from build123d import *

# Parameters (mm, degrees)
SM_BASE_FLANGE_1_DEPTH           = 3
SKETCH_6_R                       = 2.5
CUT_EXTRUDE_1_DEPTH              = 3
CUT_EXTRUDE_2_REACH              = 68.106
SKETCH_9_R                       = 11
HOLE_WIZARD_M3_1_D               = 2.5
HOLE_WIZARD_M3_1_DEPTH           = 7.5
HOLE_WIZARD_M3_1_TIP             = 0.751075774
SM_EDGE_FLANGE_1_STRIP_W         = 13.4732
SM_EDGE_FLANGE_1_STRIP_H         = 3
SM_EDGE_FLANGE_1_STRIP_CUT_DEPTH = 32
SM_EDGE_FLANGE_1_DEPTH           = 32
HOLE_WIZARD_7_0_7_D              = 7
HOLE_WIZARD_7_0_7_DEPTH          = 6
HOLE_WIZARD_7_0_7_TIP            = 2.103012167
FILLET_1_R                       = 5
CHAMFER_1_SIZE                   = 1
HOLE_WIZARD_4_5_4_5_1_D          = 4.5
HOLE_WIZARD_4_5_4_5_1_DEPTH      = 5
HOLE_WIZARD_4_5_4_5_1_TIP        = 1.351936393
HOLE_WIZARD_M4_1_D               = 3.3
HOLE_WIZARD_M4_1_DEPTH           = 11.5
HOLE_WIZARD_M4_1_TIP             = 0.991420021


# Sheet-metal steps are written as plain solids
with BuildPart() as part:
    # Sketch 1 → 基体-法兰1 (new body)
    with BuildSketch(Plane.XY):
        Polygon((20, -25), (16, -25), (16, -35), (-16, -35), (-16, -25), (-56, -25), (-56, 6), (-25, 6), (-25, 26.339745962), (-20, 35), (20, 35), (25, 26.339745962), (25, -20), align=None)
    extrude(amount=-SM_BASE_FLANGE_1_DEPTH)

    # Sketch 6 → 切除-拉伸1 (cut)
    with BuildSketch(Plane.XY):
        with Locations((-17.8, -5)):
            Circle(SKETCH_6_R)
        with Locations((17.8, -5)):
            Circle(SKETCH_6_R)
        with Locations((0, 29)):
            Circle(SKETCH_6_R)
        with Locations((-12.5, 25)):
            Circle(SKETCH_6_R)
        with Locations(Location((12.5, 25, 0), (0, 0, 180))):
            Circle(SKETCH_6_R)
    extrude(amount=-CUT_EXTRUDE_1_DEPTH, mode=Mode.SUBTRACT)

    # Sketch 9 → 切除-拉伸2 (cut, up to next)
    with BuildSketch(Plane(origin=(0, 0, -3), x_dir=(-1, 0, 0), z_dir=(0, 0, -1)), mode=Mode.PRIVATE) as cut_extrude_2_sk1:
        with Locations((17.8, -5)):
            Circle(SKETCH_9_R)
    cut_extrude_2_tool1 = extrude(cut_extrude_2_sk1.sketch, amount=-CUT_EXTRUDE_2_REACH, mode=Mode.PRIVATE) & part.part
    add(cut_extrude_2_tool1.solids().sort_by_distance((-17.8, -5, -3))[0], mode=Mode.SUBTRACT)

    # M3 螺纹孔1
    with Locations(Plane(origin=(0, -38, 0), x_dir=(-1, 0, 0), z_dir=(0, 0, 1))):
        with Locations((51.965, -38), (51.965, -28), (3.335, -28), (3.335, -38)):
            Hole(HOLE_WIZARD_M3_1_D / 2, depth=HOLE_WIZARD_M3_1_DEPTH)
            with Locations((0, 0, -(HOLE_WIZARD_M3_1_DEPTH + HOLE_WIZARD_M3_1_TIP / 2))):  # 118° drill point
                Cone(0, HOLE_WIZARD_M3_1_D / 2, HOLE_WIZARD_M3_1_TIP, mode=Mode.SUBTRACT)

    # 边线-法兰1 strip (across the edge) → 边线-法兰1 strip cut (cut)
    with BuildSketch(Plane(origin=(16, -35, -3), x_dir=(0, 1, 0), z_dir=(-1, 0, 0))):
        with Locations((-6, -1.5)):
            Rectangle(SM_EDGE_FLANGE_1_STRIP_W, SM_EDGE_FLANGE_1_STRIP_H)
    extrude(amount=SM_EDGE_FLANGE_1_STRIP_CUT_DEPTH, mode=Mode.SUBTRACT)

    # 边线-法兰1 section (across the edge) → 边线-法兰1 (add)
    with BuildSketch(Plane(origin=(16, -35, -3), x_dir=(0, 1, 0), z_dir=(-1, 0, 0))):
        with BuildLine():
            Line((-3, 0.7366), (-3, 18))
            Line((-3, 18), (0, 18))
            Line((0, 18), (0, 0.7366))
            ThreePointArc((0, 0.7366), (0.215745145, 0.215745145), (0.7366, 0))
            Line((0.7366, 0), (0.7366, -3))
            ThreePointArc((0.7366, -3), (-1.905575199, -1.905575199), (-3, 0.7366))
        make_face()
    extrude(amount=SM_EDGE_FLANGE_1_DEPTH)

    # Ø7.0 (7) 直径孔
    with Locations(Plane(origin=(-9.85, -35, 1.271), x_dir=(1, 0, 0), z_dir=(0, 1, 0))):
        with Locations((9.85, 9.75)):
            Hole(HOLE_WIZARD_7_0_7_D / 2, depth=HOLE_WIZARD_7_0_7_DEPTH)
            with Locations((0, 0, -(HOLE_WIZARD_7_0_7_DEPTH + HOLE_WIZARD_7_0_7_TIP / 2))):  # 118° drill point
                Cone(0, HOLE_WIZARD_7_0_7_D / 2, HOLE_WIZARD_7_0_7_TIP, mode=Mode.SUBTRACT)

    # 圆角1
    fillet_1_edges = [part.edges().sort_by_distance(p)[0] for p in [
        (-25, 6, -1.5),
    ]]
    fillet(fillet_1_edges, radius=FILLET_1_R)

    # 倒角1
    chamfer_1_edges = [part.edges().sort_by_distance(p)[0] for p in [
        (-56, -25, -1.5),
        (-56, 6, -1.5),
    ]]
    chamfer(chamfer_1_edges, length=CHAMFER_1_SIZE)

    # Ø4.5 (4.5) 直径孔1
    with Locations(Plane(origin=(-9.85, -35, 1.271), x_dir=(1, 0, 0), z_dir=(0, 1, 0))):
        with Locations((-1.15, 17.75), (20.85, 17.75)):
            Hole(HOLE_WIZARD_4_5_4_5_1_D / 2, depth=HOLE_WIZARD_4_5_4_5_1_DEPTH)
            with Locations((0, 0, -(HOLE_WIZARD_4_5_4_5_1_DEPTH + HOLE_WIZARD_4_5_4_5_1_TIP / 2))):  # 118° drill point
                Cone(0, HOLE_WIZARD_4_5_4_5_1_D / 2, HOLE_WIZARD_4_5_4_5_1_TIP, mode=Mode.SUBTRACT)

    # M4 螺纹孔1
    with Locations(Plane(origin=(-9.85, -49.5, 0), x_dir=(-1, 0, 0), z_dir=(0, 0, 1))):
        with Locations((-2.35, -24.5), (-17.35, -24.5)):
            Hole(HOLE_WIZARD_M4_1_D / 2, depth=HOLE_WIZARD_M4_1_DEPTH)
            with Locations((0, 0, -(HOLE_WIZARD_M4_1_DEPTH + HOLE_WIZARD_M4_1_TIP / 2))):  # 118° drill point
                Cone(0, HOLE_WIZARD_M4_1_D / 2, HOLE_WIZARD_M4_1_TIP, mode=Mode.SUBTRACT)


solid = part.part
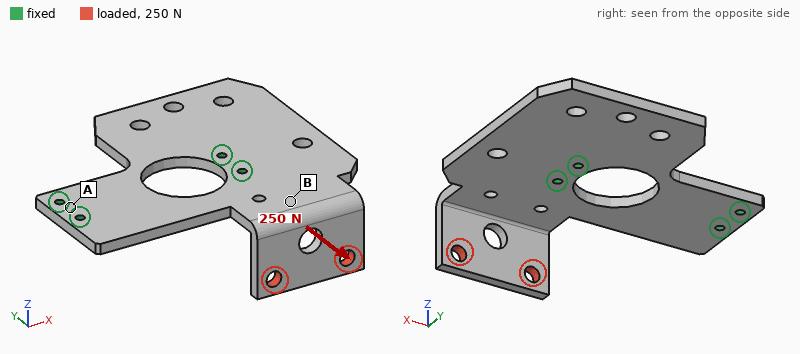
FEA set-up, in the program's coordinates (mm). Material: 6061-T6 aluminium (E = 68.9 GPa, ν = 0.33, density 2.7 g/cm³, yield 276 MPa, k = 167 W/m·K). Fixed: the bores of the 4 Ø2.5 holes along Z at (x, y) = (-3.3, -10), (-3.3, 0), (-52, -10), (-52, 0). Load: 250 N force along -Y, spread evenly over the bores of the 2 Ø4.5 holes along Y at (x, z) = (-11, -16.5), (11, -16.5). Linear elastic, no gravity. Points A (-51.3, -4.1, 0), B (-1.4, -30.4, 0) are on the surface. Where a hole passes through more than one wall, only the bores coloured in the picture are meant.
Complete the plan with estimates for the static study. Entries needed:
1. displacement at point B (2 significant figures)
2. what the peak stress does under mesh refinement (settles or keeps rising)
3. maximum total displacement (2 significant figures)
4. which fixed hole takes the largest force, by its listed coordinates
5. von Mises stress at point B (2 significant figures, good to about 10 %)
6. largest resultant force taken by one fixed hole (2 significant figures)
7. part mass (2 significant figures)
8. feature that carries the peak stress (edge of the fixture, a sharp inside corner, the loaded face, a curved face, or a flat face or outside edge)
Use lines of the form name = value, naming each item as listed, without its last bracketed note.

displacement at point B = 0.17 mm
what the peak stress does under mesh refinement = keeps rising
maximum total displacement = 0.57 mm
which fixed hole takes the largest force, by its listed coordinates = (-3.3, -10)
von Mises stress at point B = 66 MPa
largest resultant force taken by one fixed hole = 240 N
part mass = 35 g
feature that carries the peak stress = edge of the fixture
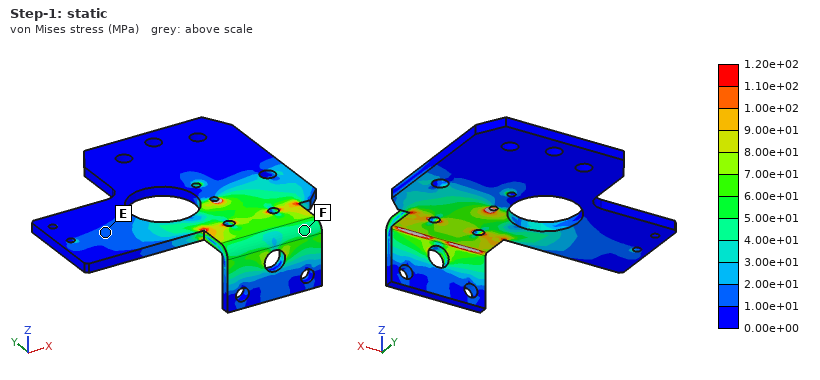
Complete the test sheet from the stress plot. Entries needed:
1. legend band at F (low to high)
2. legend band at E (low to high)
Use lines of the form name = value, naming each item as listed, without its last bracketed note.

legend band at F = 4.00e+01 to 5.00e+01 MPa
legend band at E = 1.00e+01 to 2.00e+01 MPa
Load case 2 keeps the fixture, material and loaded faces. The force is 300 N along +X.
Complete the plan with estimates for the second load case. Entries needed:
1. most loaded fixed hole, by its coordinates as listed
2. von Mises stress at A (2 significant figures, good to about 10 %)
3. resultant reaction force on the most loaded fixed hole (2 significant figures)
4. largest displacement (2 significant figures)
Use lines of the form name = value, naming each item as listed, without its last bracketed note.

most loaded fixed hole, by its coordinates as listed = (-3.3, -10)
von Mises stress at A = 11 MPa
resultant reaction force on the most loaded fixed hole = 260 N
largest displacement = 0.37 mm
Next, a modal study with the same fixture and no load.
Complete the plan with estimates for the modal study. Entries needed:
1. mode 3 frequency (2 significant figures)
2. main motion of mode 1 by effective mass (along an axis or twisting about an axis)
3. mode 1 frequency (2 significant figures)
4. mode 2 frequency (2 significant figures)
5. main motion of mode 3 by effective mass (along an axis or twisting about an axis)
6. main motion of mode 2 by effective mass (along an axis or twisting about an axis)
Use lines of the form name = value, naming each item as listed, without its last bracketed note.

mode 3 frequency = 2200 Hz
main motion of mode 1 by effective mass = twisting about X
mode 1 frequency = 1500 Hz
mode 2 frequency = 1700 Hz
main motion of mode 3 by effective mass = twisting about Y
main motion of mode 2 by effective mass = along Z
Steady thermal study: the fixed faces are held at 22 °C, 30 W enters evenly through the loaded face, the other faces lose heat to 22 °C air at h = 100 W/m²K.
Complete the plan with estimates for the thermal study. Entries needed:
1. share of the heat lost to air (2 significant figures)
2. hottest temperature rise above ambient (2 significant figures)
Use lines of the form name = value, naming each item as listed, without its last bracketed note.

share of the heat lost to air = 44 %
hottest temperature rise above ambient = 71 K
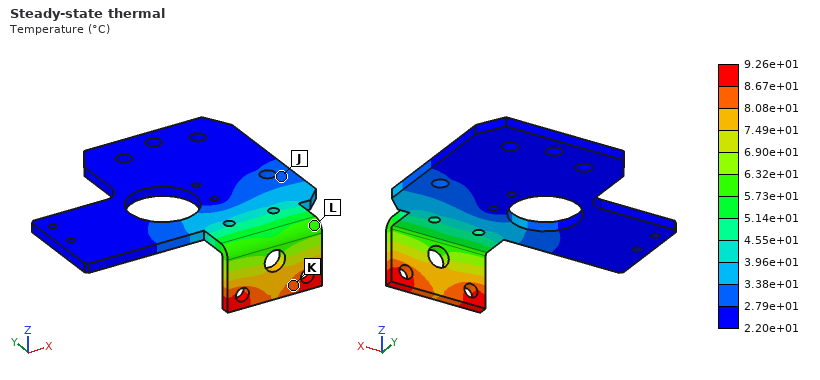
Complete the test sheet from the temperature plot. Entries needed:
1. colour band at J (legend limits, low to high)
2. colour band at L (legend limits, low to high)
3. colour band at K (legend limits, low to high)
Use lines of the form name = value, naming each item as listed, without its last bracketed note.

colour band at J = 2.79e+01 to 3.38e+01 °C
colour band at L = 5.73e+01 to 6.32e+01 °C
colour band at K = 8.08e+01 to 8.67e+01 °C
